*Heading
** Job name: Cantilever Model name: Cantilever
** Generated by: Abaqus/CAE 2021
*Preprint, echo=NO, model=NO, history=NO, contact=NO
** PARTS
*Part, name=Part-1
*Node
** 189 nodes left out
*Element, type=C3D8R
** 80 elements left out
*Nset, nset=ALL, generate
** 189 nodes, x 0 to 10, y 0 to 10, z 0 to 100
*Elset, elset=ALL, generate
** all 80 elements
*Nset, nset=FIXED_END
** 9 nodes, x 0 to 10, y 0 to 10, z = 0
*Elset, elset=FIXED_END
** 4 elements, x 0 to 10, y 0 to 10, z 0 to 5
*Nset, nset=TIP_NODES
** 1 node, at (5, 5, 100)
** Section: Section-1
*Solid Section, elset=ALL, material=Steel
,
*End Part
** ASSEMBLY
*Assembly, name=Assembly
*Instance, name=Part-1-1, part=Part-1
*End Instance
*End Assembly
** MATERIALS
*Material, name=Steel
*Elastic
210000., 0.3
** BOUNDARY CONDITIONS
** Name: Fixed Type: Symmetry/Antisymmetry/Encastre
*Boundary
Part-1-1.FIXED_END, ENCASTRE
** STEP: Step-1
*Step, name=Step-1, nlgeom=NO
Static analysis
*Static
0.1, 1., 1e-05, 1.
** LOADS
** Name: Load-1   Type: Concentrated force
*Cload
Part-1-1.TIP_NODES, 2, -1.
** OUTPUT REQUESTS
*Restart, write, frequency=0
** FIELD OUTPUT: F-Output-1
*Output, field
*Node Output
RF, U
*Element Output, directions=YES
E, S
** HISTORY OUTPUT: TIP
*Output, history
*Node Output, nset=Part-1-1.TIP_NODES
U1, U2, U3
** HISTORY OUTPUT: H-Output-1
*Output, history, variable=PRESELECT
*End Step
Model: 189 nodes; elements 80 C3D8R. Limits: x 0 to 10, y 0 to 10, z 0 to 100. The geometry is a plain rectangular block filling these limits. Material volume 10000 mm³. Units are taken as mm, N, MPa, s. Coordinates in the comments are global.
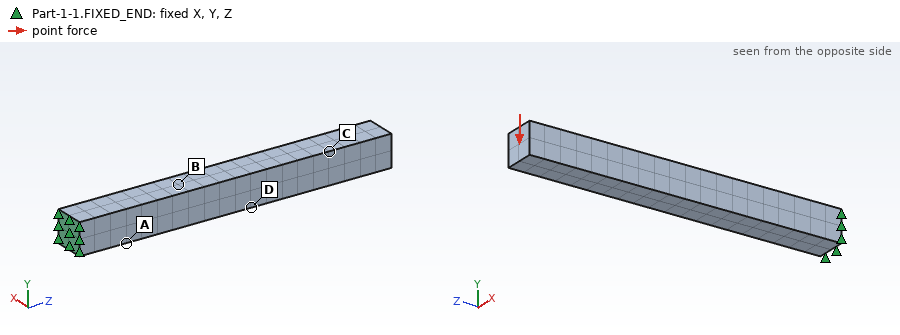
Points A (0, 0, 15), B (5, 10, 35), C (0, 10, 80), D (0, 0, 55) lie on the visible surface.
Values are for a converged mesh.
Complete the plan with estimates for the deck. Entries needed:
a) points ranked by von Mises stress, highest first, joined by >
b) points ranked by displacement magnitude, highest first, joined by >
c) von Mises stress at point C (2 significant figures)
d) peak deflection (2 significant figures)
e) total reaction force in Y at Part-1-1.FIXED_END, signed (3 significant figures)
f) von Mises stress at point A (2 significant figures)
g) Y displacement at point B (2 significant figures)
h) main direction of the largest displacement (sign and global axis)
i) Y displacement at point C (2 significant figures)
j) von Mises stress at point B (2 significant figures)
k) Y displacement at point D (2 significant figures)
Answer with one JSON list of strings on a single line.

["A > B > D > C", "C > D > B > A", "0.12 MPa", "0.0019 mm", "1.00 N", "0.51 MPa", "-3.1e-04 mm", "-Y", "-0.0013 mm", "0.39 MPa", "-7.1e-04 mm"]
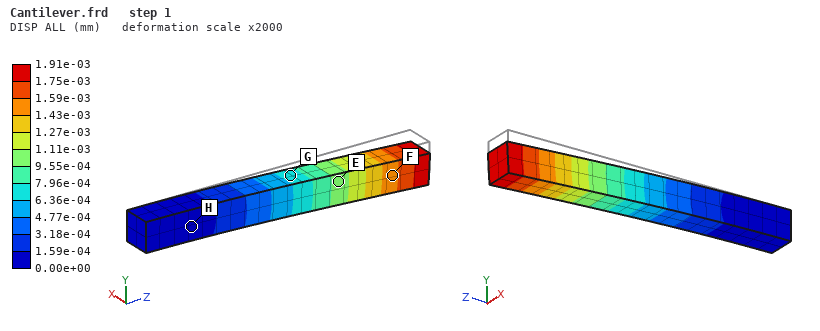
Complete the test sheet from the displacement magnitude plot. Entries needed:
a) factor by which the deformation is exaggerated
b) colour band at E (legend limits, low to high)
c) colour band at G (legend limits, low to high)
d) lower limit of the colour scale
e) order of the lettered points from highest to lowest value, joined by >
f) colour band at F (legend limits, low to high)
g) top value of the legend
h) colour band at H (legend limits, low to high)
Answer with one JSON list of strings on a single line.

["2000", "9.55e-04 to 1.11e-03 mm", "6.36e-04 to 7.96e-04 mm", "0.00e+00 mm", "F > E > G > H", "1.43e-03 to 1.59e-03 mm", "1.91e-03 mm", "0.00e+00 to 1.59e-04 mm"]
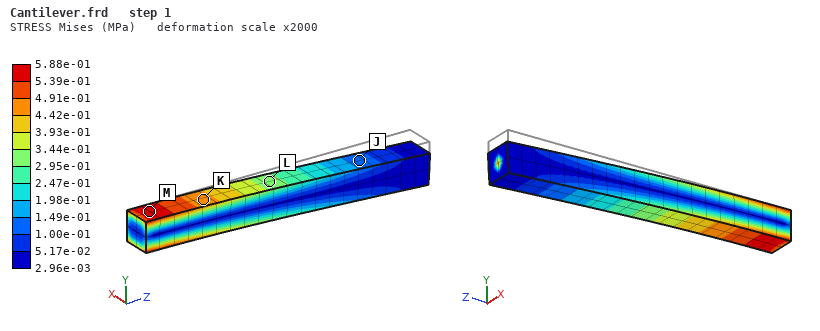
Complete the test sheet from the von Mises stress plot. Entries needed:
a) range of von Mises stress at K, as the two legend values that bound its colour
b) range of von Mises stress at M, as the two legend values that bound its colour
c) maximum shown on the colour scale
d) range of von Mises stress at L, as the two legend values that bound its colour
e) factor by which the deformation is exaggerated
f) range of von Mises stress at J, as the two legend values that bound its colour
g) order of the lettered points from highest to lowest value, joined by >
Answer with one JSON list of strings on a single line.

["4.42e-01 to 4.91e-01 MPa", "5.39e-01 to 5.88e-01 MPa", "5.88e-01 MPa", "2.95e-01 to 3.44e-01 MPa", "2000", "1.00e-01 to 1.49e-01 MPa", "M > K > L > J"]
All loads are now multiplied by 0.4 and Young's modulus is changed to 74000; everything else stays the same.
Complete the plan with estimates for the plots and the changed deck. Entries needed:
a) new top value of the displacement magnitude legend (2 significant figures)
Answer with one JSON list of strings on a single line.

["0.0022 mm"]
